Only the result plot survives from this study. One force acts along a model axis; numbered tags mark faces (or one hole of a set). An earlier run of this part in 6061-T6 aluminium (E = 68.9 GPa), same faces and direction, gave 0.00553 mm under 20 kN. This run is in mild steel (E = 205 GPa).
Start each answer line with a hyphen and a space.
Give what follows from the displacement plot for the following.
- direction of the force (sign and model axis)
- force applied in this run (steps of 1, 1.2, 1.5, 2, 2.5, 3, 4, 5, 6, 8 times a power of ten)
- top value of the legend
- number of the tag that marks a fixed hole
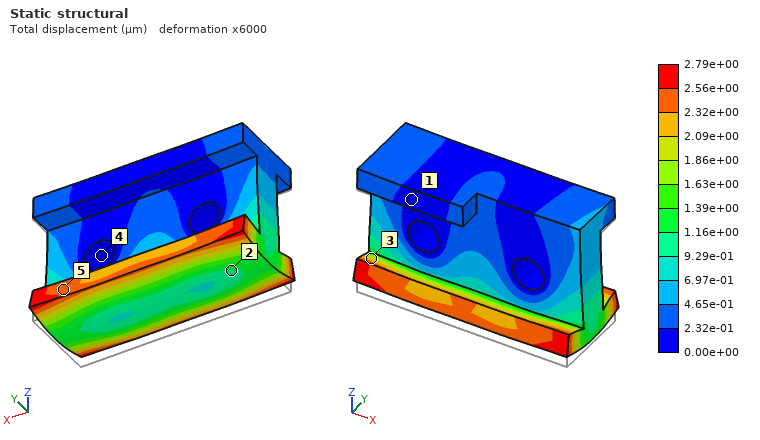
- +Z
- 30 kN
- 2.79e+00 µm
- 4
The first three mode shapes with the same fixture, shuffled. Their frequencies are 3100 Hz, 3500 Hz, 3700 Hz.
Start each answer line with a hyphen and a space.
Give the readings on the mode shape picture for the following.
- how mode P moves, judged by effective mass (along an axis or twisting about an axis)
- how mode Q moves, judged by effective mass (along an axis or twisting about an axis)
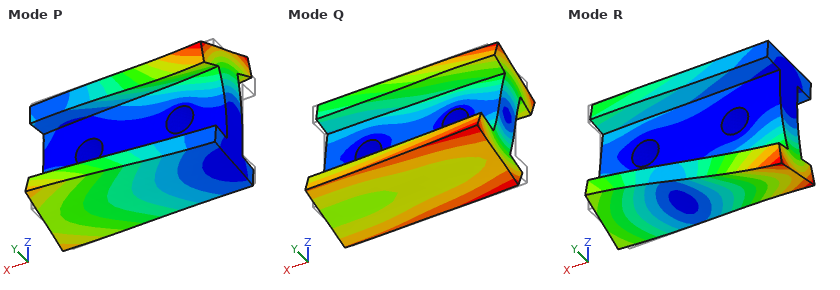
- along Y
- twisting about X
